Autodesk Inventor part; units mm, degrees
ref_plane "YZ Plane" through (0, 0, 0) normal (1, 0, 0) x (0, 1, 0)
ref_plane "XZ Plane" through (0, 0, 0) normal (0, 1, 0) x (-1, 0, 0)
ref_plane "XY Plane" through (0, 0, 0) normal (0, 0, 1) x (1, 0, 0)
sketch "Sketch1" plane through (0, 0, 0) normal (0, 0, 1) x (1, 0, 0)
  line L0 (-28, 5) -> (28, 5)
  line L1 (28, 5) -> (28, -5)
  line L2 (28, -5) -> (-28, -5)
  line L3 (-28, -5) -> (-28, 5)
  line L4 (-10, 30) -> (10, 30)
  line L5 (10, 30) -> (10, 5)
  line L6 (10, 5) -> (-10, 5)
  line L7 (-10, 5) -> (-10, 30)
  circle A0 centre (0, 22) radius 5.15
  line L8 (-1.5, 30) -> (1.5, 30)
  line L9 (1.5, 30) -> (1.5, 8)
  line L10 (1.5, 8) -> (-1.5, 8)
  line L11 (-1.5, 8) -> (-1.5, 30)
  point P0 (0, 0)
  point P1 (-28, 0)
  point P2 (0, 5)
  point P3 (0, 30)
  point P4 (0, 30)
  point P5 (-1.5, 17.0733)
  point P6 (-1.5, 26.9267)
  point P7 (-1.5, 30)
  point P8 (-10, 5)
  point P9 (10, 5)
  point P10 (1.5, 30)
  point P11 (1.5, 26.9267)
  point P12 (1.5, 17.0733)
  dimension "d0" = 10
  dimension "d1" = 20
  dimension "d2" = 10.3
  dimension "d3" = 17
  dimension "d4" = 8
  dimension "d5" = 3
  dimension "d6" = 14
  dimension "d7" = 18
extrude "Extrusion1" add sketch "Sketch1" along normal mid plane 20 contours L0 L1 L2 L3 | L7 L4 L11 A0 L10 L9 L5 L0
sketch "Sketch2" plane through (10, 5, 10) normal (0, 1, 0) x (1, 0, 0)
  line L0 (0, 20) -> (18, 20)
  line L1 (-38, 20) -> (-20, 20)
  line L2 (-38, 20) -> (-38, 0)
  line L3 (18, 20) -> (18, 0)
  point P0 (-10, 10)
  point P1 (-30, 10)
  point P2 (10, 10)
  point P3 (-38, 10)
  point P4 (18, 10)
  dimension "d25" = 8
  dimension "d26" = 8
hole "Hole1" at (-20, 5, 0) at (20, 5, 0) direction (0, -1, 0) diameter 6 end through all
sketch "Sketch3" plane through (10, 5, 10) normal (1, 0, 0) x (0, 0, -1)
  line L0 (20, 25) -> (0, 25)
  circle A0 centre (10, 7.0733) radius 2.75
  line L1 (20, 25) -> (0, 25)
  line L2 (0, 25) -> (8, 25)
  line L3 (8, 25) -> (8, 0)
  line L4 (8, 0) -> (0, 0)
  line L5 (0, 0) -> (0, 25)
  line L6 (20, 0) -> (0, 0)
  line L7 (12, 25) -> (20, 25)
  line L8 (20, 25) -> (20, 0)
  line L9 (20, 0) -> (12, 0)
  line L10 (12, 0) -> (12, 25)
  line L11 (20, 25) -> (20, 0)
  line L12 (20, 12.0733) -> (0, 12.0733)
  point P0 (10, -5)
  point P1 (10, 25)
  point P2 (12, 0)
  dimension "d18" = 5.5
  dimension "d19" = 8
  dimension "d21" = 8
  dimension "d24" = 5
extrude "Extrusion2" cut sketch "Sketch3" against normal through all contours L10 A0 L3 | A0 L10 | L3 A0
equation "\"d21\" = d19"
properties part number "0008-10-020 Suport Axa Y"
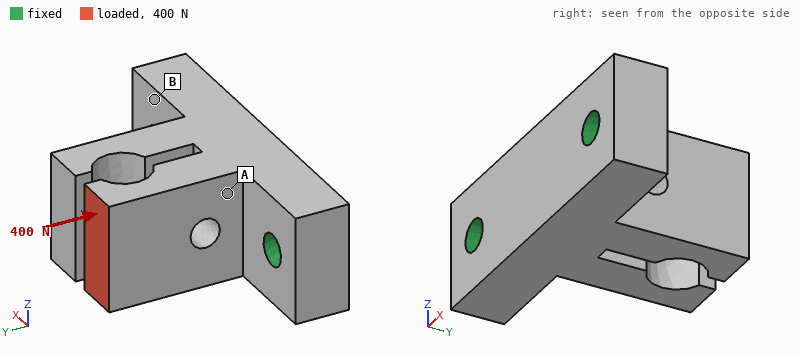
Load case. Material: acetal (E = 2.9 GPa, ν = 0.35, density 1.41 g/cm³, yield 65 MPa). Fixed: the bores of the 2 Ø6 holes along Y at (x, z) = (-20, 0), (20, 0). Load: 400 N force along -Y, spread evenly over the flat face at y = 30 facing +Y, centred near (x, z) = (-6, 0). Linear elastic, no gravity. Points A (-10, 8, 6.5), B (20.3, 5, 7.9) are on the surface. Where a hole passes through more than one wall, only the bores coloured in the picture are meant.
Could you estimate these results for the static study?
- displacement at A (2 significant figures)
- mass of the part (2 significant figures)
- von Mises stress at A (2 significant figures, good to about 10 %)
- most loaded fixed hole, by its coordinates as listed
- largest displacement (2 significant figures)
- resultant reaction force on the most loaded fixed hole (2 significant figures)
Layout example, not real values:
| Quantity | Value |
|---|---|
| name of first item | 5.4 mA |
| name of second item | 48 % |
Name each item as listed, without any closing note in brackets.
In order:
| Quantity | Value |
|---|---|
| displacement at A | 0.031 mm |
| mass of the part | 25 g |
| von Mises stress at A | 3.4 MPa |
| most loaded fixed hole, by its coordinates as listed | (-20, 0) |
| largest displacement | 0.13 mm |
| resultant reaction force on the most loaded fixed hole | 280 N |
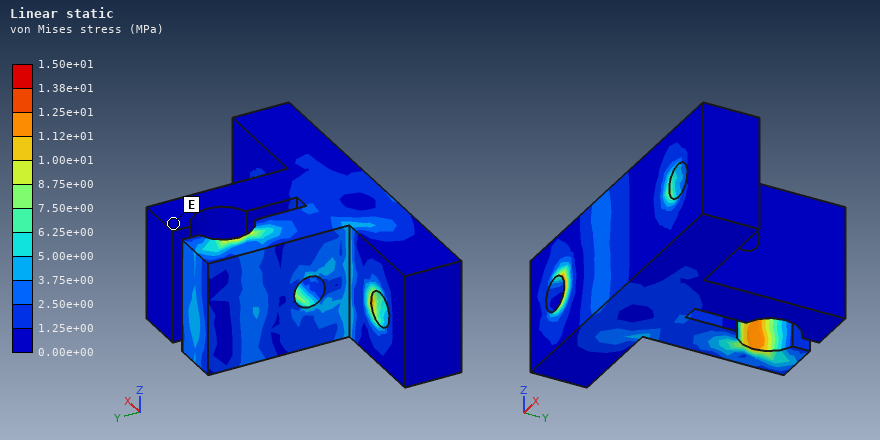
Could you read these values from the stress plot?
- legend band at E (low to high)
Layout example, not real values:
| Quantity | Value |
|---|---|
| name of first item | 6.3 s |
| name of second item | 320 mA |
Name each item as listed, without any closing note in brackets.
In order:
| Quantity | Value |
|---|---|
| legend band at E | 0.00e+00 to 1.25e+00 MPa |
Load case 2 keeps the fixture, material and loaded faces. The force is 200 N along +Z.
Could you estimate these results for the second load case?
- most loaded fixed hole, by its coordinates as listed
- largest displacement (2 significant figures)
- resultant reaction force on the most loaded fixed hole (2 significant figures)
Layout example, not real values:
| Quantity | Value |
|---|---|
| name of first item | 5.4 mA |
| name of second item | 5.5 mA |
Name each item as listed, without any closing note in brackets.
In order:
| Quantity | Value |
|---|---|
| most loaded fixed hole, by its coordinates as listed | (-20, 0) |
| largest displacement | 0.40 mm |
| resultant reaction force on the most loaded fixed hole | 130 N |
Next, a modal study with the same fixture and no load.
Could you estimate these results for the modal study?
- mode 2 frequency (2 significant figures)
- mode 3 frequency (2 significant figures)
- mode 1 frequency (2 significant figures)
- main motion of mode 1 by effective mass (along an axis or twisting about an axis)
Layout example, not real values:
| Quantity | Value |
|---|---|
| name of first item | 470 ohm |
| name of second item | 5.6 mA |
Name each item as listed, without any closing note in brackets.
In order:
| Quantity | Value |
|---|---|
| mode 2 frequency | 2500 Hz |
| mode 3 frequency | 2500 Hz |
| mode 1 frequency | 2100 Hz |
| main motion of mode 1 by effective mass | along Z |
